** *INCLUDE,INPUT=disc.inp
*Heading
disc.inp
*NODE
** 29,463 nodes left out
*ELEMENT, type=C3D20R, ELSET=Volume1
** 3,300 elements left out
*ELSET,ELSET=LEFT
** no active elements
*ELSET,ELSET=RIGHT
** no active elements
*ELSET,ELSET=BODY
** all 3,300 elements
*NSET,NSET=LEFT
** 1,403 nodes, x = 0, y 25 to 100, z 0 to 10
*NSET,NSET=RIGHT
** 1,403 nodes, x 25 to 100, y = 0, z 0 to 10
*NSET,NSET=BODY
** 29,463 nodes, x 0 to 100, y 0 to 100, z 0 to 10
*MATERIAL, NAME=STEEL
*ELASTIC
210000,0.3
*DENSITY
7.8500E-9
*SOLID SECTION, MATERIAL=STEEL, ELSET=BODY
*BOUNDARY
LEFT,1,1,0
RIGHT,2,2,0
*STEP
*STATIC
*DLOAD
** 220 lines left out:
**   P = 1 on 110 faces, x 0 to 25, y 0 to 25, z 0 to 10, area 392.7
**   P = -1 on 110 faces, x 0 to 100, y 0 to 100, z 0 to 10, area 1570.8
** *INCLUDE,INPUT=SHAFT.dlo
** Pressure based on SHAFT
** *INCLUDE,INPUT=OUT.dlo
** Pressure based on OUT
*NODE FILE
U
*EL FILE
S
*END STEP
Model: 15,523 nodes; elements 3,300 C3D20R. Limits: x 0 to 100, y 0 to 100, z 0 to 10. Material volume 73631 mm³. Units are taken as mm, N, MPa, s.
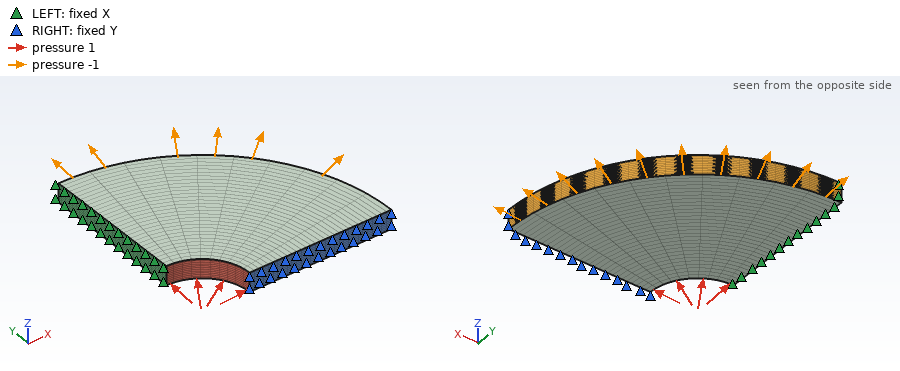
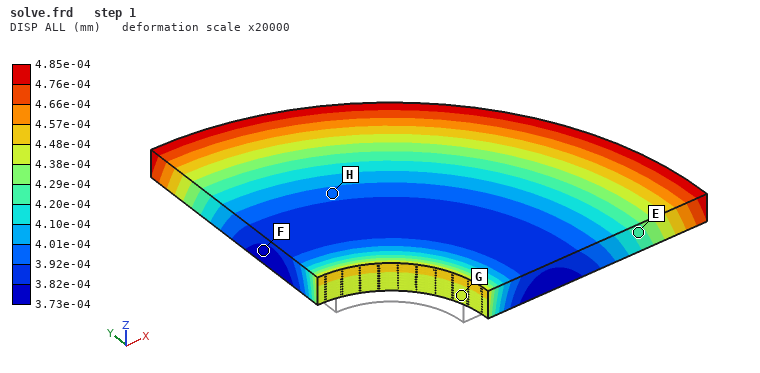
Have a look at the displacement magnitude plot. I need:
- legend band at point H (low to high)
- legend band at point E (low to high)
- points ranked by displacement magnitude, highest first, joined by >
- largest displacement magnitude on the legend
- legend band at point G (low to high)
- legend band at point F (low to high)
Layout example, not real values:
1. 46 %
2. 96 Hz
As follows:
1. 3.92e-04 to 4.01e-04 mm
2. 4.20e-04 to 4.29e-04 mm
3. G > E > H > F
4. 4.85e-04 mm
5. 4.38e-04 to 4.48e-04 mm
6. 3.73e-04 to 3.82e-04 mm
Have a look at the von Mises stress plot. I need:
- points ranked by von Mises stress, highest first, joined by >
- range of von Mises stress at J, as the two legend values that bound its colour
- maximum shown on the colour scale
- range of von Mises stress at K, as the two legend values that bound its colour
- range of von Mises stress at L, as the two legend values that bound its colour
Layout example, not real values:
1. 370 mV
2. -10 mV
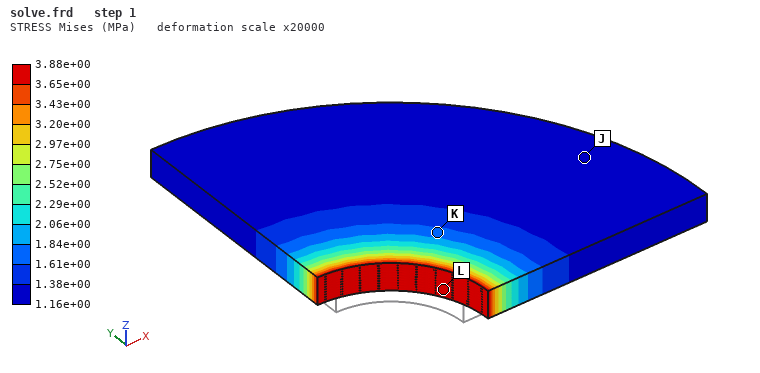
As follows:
1. L > K > J
2. 1.16e+00 to 1.38e+00 MPa
3. 3.88e+00 MPa
4. 1.61e+00 to 1.84e+00 MPa
5. 3.65e+00 to 3.88e+00 MPa
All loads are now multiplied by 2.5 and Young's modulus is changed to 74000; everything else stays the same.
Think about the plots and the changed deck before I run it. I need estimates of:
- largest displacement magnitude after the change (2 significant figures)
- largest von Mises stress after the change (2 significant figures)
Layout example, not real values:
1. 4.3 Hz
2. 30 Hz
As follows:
1. 0.0034 mm
2. 9.7 MPa
